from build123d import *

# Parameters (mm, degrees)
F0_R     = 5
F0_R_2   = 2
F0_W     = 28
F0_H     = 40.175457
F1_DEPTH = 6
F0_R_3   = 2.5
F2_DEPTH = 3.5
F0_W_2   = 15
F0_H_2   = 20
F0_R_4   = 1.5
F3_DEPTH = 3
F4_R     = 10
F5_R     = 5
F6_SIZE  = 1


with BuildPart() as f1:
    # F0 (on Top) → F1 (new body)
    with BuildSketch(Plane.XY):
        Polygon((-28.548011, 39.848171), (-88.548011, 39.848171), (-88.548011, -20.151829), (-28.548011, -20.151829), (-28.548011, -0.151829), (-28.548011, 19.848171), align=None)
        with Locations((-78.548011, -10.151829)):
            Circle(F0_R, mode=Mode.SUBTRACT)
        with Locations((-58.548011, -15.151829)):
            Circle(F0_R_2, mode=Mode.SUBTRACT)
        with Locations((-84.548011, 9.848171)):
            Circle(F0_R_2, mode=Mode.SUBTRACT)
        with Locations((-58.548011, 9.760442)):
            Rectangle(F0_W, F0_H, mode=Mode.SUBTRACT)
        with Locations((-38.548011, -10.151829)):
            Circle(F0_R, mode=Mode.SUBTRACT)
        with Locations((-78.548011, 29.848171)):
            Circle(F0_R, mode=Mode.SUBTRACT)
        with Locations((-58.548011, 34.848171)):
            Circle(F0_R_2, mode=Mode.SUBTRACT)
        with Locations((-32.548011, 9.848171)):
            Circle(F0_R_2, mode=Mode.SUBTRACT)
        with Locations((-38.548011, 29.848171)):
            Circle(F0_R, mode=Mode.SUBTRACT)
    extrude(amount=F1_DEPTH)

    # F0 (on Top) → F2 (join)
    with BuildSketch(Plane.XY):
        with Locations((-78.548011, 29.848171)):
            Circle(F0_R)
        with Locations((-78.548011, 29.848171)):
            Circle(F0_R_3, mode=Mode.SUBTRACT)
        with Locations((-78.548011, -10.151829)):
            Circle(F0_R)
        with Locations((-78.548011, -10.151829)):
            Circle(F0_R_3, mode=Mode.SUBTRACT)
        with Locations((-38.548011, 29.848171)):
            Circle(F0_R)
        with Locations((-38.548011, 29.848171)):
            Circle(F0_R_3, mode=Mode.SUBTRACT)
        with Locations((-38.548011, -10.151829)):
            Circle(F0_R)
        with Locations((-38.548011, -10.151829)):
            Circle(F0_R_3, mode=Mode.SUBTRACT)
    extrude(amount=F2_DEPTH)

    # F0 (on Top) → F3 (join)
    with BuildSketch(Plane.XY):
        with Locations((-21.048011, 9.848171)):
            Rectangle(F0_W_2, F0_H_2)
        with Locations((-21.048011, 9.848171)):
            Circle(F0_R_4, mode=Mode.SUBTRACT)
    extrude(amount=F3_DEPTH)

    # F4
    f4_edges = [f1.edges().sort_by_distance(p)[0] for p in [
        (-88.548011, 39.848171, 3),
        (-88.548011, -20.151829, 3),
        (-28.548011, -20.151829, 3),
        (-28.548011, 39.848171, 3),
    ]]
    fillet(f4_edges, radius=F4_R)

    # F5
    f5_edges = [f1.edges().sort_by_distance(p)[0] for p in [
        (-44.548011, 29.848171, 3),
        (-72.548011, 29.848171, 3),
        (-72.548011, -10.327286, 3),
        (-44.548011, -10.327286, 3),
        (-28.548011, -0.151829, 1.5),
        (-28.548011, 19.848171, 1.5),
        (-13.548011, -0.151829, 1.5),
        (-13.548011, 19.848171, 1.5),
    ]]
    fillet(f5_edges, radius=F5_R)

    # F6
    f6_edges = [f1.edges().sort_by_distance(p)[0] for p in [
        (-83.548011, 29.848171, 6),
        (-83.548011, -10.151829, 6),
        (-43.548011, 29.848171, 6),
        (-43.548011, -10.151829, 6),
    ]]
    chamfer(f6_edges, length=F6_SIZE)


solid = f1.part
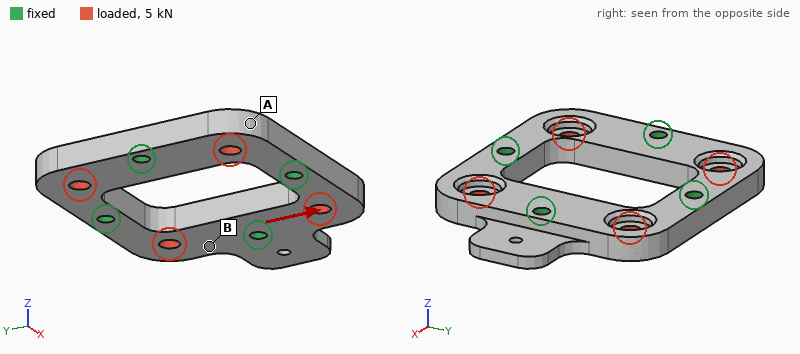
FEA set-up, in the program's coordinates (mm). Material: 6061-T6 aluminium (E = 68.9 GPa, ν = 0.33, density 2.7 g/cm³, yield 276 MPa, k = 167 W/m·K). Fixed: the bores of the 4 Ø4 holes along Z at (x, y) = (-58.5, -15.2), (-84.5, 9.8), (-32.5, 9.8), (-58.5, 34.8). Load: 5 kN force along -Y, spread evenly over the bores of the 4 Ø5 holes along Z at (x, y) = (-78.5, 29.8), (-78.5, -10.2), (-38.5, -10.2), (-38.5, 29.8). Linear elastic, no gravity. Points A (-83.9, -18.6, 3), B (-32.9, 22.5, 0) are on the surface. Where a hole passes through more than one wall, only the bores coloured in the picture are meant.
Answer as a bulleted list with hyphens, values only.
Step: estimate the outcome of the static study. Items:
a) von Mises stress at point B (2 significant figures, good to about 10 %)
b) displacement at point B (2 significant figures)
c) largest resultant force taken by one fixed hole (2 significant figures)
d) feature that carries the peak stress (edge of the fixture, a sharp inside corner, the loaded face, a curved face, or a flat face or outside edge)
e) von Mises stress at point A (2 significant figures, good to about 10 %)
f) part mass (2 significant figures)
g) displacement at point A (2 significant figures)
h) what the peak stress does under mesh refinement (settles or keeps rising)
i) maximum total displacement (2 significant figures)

- 20 MPa
- 4.7 µm
- 2.1 kN
- edge of the fixture
- 7.2 MPa
- 38 g
- 11 µm
- keeps rising
- 12 µm
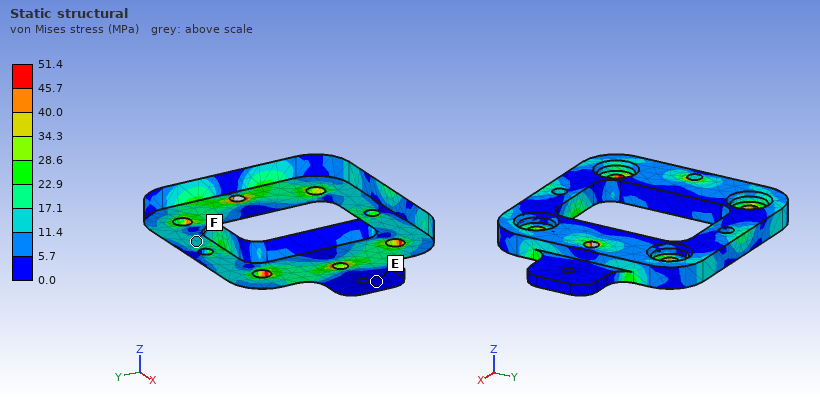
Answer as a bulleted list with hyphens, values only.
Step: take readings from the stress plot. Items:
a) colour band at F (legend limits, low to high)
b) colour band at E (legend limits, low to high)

- 11.4 to 17.1 MPa
- 0.0 to 5.7 MPa
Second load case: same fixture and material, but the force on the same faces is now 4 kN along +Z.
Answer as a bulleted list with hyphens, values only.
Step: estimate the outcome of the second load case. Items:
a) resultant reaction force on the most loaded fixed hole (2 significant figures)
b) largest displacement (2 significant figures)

- 1.1 kN
- 68 µm
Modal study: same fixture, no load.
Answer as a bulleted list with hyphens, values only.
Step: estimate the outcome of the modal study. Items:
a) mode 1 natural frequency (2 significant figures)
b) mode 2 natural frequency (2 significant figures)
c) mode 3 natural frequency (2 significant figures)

- 9600 Hz
- 10 kHz
- 11 kHz
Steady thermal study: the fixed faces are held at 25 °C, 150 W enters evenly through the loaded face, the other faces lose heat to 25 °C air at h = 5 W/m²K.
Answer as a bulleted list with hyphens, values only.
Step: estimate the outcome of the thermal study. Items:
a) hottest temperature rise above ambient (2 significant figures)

- 38 K
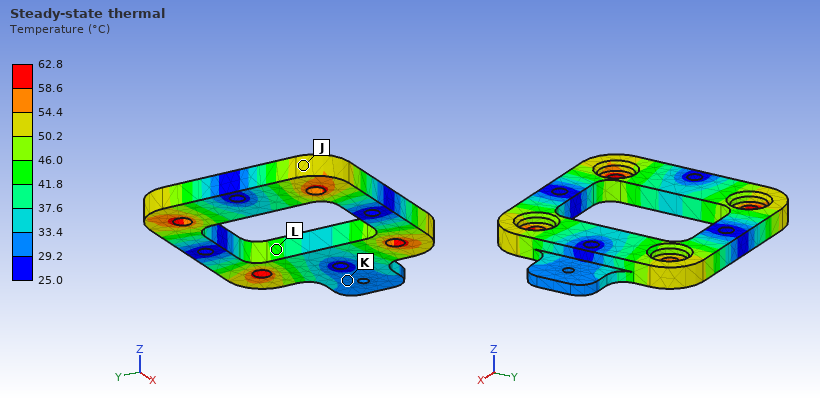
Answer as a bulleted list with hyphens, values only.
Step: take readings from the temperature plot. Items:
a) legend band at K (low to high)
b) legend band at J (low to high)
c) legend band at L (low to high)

- 29.2 to 33.4 °C
- 50.2 to 54.4 °C
- 41.8 to 46.0 °C
